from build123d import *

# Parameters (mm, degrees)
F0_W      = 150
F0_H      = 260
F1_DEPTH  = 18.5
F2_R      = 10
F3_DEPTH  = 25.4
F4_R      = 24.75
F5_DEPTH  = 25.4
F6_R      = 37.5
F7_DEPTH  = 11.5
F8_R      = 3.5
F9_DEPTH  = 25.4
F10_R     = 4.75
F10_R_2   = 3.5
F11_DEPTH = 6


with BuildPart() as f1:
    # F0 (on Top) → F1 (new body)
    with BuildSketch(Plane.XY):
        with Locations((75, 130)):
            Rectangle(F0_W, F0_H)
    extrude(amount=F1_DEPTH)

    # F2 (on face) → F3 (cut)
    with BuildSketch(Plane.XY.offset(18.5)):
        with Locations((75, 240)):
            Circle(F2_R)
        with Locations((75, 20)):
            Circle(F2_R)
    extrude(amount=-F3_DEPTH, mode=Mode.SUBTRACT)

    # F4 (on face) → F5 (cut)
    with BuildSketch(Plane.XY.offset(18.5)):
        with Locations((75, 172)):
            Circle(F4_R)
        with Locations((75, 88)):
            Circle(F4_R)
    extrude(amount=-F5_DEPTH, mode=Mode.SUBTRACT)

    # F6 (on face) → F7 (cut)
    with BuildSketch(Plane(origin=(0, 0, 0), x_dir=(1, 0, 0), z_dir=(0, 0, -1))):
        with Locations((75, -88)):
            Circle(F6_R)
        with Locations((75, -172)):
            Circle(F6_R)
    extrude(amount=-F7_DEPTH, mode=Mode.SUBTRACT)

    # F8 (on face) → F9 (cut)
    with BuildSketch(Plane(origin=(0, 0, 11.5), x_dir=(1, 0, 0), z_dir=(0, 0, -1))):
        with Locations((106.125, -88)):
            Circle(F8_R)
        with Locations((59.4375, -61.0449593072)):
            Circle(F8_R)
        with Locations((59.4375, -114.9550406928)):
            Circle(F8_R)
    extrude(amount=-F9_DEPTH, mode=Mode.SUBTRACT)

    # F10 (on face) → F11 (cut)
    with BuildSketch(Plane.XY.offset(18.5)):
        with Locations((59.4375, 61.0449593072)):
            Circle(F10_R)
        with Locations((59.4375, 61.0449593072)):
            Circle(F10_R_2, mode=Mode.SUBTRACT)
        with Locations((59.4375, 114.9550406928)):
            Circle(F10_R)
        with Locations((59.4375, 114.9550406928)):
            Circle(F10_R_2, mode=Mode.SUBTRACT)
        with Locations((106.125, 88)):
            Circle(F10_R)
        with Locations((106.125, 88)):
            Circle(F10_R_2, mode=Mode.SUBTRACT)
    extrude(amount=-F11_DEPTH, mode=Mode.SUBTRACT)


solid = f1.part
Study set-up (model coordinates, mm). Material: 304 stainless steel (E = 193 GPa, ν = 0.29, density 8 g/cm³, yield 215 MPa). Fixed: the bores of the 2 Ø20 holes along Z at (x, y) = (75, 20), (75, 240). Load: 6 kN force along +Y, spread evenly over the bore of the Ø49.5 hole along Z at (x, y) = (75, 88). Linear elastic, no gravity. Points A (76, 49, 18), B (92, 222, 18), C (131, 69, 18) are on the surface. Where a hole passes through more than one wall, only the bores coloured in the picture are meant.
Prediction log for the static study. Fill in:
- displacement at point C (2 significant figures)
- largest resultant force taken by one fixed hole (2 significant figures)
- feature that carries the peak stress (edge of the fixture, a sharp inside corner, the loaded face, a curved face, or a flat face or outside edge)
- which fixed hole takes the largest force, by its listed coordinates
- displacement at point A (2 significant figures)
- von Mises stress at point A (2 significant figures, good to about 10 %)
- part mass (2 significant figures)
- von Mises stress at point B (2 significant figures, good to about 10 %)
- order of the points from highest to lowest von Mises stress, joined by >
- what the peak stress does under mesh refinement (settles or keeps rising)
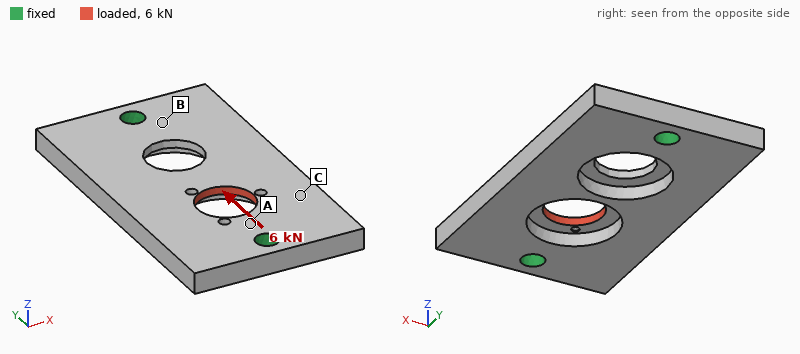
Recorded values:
1.8 µm
3.9 kN
a sharp inside corner
(75, 20)
0.94 µm
8.7 MPa
4.6 kg
2.5 MPa
A > B > C
keeps rising
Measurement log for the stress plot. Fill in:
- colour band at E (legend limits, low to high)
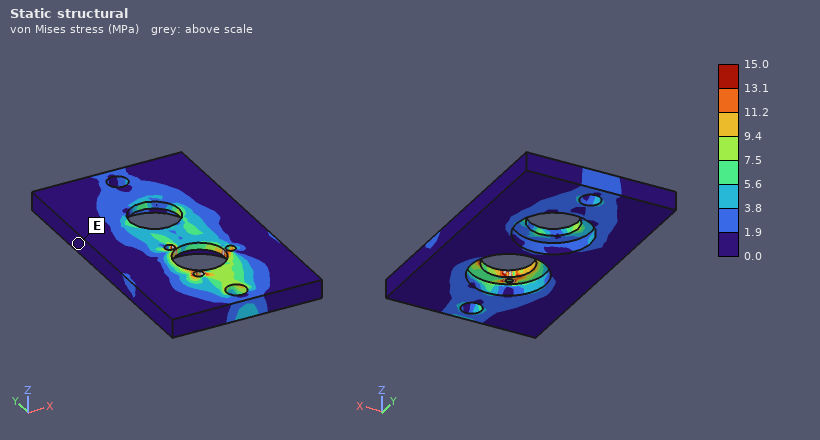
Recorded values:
0.0 to 1.9 MPa
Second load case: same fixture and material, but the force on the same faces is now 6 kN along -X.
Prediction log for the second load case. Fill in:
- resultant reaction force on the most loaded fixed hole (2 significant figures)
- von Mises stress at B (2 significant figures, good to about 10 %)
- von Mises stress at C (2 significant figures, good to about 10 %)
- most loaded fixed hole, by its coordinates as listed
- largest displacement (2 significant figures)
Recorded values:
4.2 kN
4.2 MPa
3.8 MPa
(75, 20)
5.8 µm
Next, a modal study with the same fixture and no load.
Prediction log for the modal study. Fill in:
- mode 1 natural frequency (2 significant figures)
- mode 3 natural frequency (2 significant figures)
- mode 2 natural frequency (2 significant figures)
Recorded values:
1400 Hz
2700 Hz
1400 Hz
